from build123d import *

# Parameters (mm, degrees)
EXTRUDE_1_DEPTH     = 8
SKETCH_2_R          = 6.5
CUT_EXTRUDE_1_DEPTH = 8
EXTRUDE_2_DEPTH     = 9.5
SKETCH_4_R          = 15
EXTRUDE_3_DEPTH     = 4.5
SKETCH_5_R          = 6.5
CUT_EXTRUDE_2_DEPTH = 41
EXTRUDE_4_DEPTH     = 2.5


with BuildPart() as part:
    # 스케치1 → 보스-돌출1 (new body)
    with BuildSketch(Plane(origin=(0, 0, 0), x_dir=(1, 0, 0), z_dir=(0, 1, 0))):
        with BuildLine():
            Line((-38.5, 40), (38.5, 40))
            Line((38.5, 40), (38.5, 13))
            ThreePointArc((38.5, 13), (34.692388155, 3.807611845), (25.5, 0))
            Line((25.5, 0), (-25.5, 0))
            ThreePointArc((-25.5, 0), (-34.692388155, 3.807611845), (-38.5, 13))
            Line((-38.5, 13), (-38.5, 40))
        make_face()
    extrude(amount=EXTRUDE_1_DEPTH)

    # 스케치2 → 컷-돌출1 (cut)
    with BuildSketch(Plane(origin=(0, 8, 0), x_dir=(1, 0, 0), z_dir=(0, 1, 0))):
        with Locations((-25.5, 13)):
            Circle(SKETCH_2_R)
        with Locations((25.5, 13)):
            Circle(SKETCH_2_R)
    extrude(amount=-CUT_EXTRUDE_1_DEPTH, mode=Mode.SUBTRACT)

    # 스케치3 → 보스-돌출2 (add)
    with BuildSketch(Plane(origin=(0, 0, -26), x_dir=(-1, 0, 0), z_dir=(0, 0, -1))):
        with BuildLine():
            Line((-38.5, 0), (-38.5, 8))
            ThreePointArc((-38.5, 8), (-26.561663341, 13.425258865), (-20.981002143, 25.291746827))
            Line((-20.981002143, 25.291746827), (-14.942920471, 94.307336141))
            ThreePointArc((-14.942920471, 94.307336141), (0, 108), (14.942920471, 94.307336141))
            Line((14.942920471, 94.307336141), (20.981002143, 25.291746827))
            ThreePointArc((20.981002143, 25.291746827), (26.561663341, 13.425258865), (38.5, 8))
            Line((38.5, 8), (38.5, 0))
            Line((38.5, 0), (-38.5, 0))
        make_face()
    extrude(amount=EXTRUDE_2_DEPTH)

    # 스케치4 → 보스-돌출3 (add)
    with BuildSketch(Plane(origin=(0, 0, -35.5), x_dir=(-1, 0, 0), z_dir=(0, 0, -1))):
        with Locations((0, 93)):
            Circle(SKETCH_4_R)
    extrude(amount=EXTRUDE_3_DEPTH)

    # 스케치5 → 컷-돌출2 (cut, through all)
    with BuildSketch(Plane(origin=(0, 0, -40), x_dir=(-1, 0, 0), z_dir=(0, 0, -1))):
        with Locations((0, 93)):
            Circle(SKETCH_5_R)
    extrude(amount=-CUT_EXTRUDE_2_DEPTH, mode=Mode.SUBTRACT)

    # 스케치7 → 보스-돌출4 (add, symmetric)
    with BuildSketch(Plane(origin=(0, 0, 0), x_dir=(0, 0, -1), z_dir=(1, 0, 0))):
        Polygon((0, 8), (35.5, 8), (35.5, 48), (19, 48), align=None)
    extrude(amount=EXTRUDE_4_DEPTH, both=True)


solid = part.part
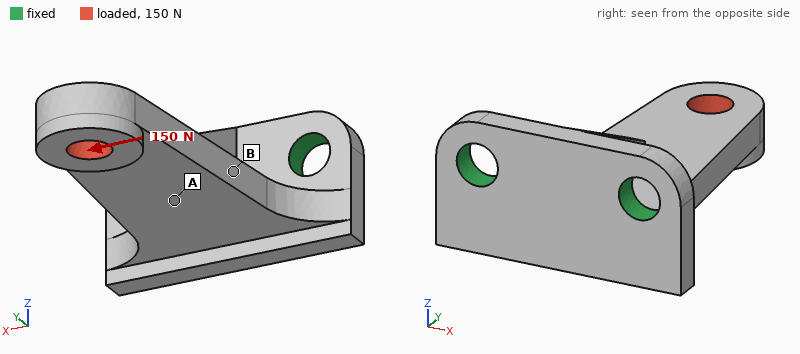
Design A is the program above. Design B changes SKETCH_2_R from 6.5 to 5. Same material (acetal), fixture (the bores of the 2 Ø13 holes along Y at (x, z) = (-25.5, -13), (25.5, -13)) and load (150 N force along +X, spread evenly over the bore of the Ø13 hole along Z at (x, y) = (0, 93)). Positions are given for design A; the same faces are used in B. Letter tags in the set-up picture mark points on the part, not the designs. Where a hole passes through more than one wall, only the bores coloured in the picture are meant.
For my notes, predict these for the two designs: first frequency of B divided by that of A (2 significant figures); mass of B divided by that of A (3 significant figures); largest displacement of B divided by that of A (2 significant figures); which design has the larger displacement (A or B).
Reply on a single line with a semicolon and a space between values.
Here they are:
0.94; 1.01; 1.1; B
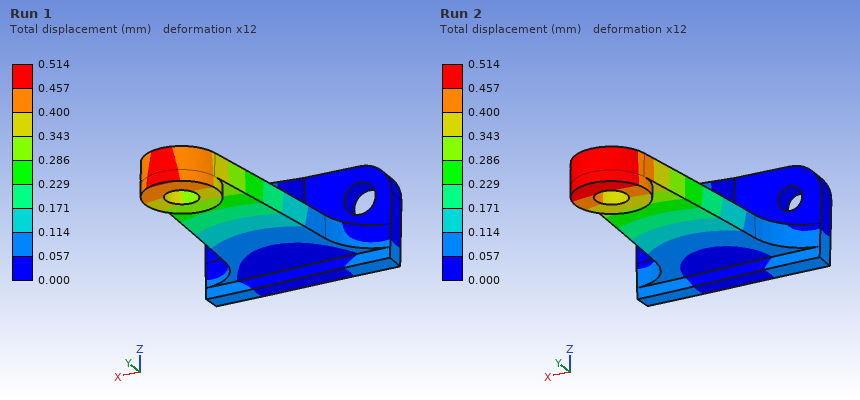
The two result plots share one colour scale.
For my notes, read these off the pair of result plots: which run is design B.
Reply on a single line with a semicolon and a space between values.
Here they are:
Run 2
